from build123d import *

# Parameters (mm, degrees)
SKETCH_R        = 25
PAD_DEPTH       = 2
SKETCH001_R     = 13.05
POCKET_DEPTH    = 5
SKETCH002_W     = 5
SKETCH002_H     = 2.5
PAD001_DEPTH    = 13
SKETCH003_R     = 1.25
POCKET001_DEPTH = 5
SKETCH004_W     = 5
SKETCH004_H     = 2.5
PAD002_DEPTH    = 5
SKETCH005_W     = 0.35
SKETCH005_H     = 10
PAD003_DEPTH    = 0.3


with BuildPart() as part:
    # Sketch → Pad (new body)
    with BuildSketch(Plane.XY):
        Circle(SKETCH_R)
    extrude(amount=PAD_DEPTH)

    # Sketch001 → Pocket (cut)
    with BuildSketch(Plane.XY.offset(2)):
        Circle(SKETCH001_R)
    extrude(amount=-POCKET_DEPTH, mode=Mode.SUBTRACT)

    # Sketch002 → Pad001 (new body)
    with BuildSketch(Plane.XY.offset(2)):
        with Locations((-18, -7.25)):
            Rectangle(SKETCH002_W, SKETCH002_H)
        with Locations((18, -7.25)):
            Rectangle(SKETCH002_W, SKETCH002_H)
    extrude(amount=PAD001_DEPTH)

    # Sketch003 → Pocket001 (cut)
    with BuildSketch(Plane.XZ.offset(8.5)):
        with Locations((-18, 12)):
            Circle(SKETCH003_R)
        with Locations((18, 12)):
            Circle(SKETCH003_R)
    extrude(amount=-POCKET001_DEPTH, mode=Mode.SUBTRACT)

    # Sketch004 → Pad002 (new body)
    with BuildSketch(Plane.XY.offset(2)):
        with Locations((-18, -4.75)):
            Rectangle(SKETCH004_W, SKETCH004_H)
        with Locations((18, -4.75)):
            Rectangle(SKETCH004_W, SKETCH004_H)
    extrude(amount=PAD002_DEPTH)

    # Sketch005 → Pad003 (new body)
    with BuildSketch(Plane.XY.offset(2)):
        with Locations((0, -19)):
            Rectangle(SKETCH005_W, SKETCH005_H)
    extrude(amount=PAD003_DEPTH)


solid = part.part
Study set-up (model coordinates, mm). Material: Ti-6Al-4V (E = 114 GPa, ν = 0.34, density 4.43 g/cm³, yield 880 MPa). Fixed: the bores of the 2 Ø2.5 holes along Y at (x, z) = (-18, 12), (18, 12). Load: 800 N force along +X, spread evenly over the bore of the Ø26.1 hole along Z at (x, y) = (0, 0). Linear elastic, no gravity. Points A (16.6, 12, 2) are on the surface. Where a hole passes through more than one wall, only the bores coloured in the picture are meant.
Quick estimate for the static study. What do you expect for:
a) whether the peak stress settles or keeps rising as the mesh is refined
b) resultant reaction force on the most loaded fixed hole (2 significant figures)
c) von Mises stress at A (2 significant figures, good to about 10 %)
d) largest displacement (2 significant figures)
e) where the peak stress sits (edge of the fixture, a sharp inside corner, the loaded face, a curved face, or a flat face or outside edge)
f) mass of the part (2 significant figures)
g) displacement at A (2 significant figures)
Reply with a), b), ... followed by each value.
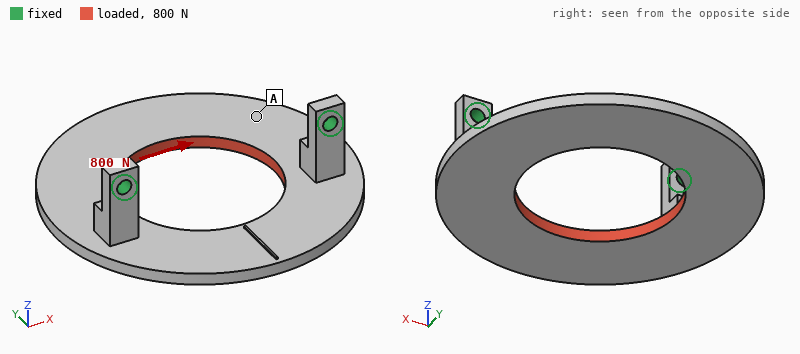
a) keeps rising
b) 430 N
c) 36 MPa
d) 0.12 mm
e) edge of the fixture
f) 15 g
g) 0.11 mm
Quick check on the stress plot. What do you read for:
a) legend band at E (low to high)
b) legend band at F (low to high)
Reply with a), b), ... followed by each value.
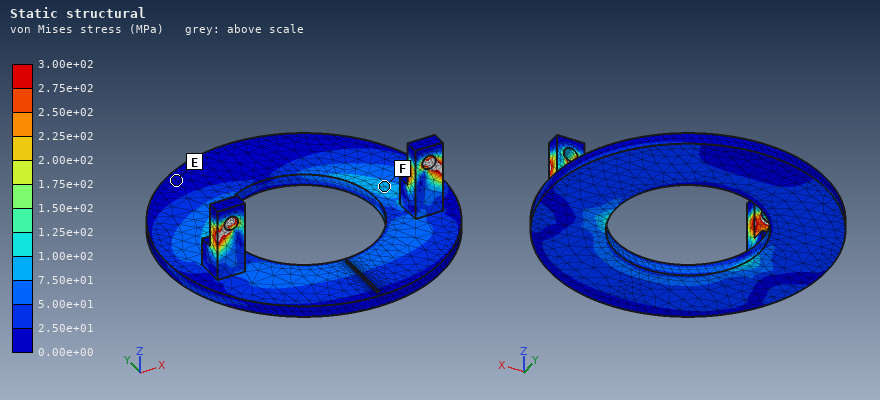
a) 0.00e+00 to 2.50e+01 MPa
b) 7.50e+01 to 1.00e+02 MPa
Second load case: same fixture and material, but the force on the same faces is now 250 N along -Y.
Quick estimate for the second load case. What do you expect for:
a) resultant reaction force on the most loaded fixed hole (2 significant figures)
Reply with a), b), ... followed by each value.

a) 130 N
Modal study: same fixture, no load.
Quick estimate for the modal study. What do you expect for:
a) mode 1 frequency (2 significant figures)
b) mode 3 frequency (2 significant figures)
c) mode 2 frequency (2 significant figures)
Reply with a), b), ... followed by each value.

a) 1100 Hz
b) 3000 Hz
c) 2700 Hz
